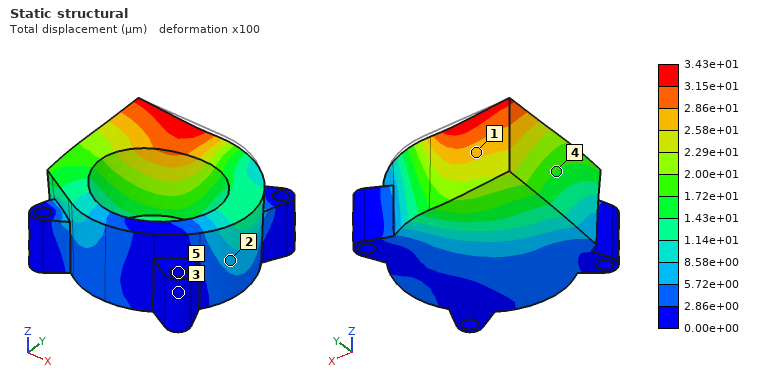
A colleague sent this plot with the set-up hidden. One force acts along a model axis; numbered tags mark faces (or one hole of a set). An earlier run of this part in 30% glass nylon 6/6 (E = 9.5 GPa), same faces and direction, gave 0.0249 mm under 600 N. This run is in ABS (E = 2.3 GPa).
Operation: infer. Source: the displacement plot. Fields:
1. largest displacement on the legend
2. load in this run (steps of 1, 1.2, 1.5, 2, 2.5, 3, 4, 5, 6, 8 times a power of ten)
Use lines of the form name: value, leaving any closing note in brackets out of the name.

largest displacement on the legend: 3.43e+01 µm
load in this run: 200 N
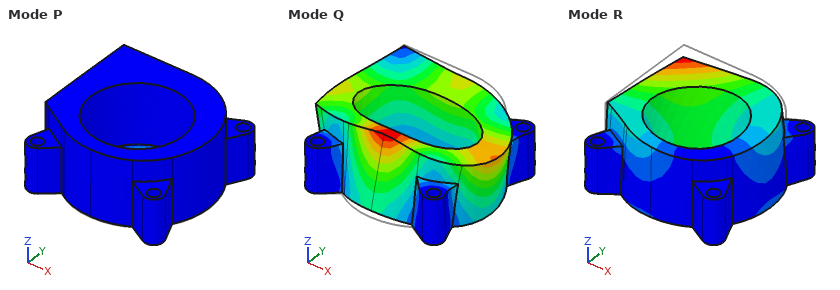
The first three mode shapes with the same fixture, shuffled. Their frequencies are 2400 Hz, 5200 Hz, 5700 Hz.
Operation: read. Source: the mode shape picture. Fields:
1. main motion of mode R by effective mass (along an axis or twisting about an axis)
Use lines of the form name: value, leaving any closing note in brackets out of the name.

main motion of mode R by effective mass: along Z
